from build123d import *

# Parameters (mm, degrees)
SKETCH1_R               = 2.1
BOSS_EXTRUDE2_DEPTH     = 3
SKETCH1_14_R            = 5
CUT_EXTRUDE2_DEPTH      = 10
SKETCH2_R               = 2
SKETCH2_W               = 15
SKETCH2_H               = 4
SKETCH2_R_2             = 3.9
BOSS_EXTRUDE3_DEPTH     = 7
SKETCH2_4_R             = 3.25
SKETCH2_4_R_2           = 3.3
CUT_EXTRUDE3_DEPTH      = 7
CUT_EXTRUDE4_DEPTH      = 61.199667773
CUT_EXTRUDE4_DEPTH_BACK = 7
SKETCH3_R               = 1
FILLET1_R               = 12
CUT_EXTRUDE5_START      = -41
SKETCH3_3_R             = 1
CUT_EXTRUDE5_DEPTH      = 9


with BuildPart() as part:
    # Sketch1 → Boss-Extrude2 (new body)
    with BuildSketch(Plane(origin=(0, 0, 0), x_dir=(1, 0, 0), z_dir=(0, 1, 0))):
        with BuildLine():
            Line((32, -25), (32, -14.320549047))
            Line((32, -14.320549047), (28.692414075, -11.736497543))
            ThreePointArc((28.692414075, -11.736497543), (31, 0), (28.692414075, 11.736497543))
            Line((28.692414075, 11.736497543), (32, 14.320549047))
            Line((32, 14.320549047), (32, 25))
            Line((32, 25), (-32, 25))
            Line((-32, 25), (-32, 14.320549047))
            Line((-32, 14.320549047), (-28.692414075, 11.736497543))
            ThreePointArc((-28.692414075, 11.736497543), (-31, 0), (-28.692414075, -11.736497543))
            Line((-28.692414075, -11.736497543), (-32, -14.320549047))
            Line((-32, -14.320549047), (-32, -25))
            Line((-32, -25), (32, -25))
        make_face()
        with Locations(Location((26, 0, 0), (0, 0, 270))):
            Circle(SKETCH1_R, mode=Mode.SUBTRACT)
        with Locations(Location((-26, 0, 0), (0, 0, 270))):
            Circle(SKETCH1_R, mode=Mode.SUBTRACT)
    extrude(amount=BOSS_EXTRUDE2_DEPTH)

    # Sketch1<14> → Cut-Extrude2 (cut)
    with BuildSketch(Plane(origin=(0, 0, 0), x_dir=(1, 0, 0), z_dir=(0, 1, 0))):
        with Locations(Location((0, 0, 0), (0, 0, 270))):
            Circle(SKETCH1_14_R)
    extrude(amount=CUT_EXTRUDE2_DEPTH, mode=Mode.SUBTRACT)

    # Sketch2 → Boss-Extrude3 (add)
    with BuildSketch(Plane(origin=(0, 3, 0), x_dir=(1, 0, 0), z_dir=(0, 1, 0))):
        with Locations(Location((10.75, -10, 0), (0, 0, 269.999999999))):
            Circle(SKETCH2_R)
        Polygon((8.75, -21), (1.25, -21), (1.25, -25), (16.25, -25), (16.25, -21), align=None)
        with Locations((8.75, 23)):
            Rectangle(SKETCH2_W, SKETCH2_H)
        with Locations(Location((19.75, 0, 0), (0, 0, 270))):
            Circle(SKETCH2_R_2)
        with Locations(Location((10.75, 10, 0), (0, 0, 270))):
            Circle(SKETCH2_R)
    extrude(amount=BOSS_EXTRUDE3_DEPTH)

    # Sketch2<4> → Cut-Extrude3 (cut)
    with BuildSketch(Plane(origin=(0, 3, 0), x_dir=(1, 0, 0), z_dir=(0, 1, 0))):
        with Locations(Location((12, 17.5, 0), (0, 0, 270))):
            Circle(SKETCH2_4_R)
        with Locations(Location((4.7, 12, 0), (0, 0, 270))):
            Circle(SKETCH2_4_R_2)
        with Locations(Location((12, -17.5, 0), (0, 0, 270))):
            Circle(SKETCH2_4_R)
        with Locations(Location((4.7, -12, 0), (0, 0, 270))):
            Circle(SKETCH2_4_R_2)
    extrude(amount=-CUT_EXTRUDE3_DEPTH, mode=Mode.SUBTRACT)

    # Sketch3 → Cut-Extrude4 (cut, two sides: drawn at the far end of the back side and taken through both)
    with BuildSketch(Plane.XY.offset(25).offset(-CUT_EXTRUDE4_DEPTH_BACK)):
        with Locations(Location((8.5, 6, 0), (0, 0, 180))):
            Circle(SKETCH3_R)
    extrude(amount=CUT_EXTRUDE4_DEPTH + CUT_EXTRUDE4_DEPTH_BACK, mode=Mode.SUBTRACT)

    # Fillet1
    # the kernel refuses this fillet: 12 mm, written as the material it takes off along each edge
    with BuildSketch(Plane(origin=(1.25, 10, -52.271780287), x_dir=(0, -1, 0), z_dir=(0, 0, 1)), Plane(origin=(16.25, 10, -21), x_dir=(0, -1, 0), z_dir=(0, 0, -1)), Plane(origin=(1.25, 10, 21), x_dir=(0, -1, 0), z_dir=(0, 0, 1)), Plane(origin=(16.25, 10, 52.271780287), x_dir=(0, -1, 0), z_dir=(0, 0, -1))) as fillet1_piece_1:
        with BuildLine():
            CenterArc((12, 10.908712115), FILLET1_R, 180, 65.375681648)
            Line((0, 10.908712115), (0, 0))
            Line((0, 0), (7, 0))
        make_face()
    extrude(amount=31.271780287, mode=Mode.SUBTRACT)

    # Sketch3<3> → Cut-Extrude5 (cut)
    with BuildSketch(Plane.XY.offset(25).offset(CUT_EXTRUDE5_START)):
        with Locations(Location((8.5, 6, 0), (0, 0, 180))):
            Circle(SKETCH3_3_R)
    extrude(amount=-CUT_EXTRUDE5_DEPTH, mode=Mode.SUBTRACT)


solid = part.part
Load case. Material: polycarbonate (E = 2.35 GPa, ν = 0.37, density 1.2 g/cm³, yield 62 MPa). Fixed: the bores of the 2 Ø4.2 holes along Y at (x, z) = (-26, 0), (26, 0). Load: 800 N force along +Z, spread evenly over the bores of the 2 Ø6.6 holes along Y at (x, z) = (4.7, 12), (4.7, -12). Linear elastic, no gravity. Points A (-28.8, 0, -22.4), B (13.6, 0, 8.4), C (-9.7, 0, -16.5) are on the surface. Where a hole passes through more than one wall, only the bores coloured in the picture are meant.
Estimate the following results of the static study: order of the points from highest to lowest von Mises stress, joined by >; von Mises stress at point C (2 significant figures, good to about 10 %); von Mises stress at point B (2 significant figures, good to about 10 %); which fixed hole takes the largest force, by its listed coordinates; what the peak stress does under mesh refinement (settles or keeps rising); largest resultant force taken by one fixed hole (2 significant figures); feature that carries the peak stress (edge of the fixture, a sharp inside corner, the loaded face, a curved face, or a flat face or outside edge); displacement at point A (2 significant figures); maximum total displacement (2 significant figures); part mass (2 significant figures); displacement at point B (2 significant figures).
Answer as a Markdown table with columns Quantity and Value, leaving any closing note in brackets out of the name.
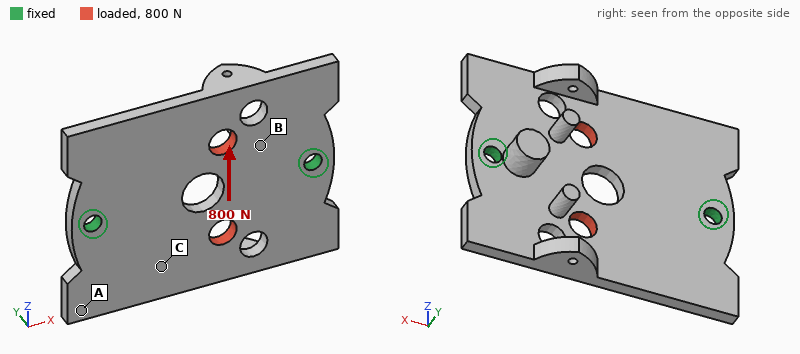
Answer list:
| Quantity | Value |
|---|---|
| order of the points from highest to lowest von Mises stress, joined by > | B > C > A |
| von Mises stress at point C | 4.0 MPa |
| von Mises stress at point B | 8.0 MPa |
| which fixed hole takes the largest force, by its listed coordinates | (26, 0) |
| what the peak stress does under mesh refinement | keeps rising |
| largest resultant force taken by one fixed hole | 480 N |
| feature that carries the peak stress | edge of the fixture |
| displacement at point A | 0.051 mm |
| maximum total displacement | 0.16 mm |
| part mass | 11 g |
| displacement at point B | 0.098 mm |
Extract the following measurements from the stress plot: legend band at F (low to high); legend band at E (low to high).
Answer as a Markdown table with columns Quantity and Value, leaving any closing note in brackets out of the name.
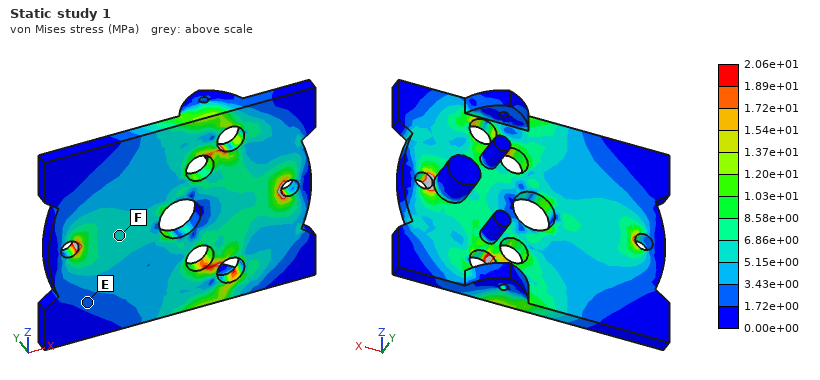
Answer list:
| Quantity | Value |
|---|---|
| legend band at F | 5.15e+00 to 6.86e+00 MPa |
| legend band at E | 1.72e+00 to 3.43e+00 MPa |
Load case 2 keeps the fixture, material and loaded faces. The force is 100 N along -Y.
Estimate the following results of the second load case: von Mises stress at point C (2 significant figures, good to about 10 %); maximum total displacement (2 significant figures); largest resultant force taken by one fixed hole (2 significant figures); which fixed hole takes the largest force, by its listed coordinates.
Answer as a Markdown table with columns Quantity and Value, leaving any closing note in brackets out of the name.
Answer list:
| Quantity | Value |
|---|---|
| von Mises stress at point C | 2.2 MPa |
| maximum total displacement | 0.55 mm |
| largest resultant force taken by one fixed hole | 63 N |
| which fixed hole takes the largest force, by its listed coordinates | (26, 0) |
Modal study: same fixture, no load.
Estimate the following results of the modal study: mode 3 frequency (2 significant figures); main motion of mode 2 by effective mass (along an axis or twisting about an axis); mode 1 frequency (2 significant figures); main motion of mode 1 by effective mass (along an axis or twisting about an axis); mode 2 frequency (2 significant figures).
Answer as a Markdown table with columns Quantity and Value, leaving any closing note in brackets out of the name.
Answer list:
| Quantity | Value |
|---|---|
| mode 3 frequency | 1400 Hz |
| main motion of mode 2 by effective mass | along Y |
| mode 1 frequency | 680 Hz |
| main motion of mode 1 by effective mass | twisting about X |
| mode 2 frequency | 890 Hz |
